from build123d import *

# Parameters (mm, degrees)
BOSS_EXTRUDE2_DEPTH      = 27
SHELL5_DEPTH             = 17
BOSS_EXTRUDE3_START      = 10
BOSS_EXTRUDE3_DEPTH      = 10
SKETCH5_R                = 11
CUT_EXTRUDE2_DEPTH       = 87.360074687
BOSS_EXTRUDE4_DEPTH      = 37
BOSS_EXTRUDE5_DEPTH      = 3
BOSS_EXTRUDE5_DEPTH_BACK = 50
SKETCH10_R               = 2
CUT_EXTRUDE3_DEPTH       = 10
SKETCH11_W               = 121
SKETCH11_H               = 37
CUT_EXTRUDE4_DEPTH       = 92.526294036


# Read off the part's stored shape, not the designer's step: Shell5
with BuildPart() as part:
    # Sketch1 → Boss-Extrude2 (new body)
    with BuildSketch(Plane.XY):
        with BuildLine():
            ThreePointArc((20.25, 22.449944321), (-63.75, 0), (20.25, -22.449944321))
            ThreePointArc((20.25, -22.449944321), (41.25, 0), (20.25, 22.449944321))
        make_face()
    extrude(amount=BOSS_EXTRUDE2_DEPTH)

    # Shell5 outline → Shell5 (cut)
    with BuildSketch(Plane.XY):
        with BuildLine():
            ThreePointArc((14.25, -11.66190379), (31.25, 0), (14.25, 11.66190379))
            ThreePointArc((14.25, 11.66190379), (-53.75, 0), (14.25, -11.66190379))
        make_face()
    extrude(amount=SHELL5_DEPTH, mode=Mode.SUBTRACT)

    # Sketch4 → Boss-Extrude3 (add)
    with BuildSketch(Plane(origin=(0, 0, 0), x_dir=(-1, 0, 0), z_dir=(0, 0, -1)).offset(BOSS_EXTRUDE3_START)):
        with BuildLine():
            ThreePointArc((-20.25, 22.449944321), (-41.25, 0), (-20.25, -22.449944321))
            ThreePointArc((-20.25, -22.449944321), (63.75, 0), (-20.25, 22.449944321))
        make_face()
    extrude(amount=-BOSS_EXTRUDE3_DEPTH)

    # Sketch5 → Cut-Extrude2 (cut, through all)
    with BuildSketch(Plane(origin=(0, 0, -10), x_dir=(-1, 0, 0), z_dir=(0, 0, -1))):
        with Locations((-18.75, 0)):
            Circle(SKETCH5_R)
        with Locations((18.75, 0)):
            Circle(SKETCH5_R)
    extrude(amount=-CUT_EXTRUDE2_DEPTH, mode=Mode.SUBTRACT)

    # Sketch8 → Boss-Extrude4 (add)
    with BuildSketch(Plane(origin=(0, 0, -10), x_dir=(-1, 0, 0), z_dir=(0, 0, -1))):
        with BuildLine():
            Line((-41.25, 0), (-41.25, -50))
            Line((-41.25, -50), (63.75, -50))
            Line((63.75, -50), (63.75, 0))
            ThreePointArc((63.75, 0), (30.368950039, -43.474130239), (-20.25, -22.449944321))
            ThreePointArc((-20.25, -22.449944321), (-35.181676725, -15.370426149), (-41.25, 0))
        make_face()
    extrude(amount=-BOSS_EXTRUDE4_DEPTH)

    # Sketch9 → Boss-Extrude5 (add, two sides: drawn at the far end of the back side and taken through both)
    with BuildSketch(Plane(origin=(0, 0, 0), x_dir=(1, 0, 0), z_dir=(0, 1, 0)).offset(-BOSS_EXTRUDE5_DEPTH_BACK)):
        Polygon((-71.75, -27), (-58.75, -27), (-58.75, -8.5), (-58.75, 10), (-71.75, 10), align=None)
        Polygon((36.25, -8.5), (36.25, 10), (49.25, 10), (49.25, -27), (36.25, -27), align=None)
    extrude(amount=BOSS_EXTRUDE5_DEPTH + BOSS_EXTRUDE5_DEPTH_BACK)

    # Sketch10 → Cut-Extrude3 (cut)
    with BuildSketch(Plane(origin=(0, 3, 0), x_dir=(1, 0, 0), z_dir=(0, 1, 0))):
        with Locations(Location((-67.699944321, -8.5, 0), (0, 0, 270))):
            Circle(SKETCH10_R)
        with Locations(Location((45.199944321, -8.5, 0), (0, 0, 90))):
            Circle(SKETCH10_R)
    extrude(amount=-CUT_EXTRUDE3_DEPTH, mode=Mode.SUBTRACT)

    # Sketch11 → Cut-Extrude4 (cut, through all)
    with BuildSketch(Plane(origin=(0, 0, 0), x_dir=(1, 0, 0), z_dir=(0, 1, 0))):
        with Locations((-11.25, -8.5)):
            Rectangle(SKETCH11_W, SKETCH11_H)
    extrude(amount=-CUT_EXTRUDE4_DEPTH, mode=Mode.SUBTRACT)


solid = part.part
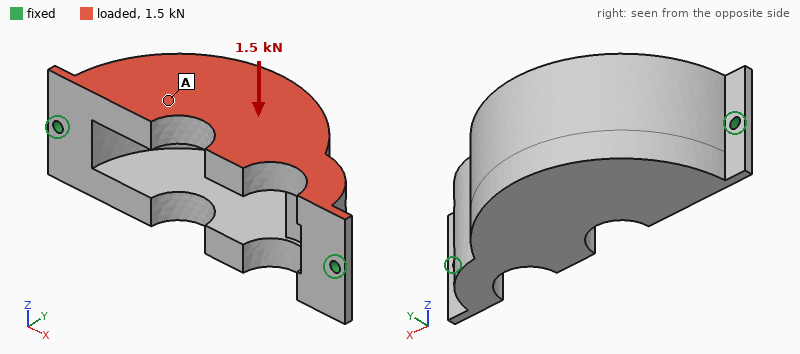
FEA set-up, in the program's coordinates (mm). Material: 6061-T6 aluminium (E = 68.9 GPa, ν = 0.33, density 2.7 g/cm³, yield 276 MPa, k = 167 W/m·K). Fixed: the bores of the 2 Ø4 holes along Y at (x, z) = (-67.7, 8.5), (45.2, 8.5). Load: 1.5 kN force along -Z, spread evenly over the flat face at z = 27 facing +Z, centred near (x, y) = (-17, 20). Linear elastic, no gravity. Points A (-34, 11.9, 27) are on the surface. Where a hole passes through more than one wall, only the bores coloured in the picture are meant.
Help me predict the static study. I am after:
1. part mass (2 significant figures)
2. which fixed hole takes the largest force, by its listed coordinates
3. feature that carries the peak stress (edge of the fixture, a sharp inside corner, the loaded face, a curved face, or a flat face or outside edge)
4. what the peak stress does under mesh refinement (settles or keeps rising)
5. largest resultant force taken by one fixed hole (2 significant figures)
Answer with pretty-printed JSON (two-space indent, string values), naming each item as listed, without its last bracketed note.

{
  "part mass": "230 g",
  "which fixed hole takes the largest force, by its listed coordinates": "(-67.7, 8.5)",
  "feature that carries the peak stress": "edge of the fixture",
  "what the peak stress does under mesh refinement": "keeps rising",
  "largest resultant force taken by one fixed hole": "810 N"
}
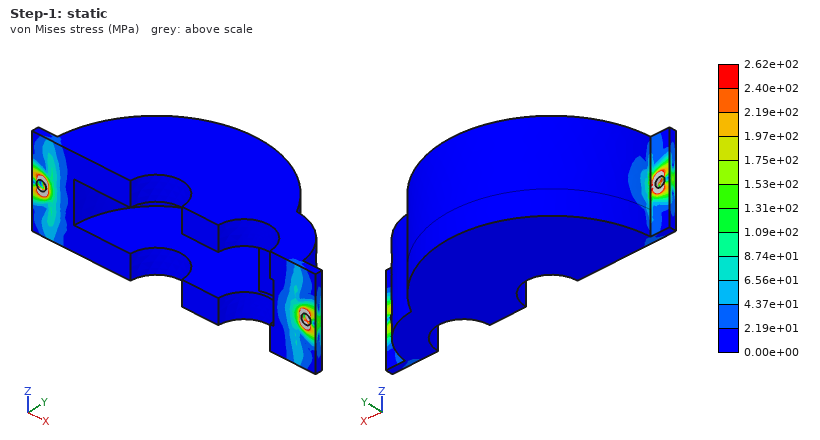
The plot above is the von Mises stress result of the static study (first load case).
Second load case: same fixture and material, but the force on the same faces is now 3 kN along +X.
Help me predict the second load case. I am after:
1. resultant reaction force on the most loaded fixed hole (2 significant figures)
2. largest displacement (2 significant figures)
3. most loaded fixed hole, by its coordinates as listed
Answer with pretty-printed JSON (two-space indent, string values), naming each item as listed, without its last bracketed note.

{
  "resultant reaction force on the most loaded fixed hole": "1.9 kN",
  "largest displacement": "23 µm",
  "most loaded fixed hole, by its coordinates as listed": "(-67.7, 8.5)"
}
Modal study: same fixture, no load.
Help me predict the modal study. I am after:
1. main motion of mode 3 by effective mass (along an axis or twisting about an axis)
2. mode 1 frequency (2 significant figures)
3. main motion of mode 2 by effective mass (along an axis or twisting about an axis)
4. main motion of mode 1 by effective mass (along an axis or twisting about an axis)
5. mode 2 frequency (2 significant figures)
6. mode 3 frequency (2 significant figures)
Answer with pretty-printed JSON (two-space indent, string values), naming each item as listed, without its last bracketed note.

{
  "main motion of mode 3 by effective mass": "along X",
  "mode 1 frequency": "630 Hz",
  "main motion of mode 2 by effective mass": "along Y",
  "main motion of mode 1 by effective mass": "along Z",
  "mode 2 frequency": "3800 Hz",
  "mode 3 frequency": "5600 Hz"
}
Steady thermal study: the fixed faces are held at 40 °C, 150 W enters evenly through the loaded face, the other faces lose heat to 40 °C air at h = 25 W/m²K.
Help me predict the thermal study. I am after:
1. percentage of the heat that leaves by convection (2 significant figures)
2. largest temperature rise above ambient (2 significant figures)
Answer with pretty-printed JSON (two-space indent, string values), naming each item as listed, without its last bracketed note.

{
  "percentage of the heat that leaves by convection": "18 %",
  "largest temperature rise above ambient": "78 K"
}
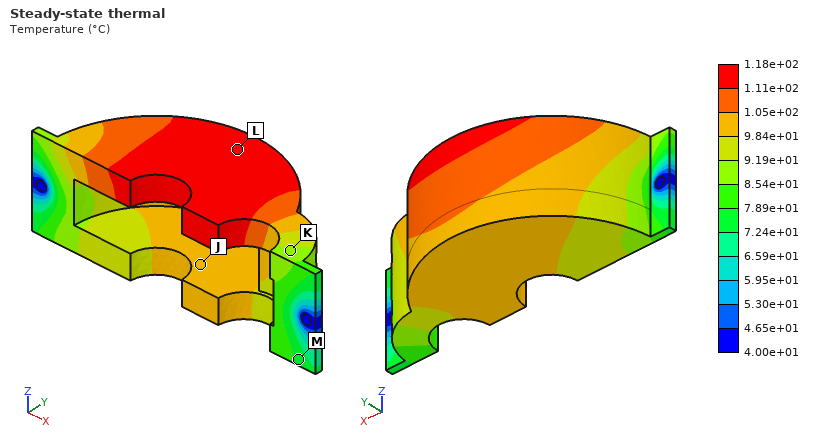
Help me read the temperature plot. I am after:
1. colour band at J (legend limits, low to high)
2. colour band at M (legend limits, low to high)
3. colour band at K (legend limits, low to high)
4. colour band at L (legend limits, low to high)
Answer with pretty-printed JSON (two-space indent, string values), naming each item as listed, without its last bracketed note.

{
  "colour band at J": "9.84e+01 to 1.05e+02 °C",
  "colour band at M": "7.24e+01 to 7.89e+01 °C",
  "colour band at K": "8.54e+01 to 9.19e+01 °C",
  "colour band at L": "1.11e+02 to 1.18e+02 °C"
}
